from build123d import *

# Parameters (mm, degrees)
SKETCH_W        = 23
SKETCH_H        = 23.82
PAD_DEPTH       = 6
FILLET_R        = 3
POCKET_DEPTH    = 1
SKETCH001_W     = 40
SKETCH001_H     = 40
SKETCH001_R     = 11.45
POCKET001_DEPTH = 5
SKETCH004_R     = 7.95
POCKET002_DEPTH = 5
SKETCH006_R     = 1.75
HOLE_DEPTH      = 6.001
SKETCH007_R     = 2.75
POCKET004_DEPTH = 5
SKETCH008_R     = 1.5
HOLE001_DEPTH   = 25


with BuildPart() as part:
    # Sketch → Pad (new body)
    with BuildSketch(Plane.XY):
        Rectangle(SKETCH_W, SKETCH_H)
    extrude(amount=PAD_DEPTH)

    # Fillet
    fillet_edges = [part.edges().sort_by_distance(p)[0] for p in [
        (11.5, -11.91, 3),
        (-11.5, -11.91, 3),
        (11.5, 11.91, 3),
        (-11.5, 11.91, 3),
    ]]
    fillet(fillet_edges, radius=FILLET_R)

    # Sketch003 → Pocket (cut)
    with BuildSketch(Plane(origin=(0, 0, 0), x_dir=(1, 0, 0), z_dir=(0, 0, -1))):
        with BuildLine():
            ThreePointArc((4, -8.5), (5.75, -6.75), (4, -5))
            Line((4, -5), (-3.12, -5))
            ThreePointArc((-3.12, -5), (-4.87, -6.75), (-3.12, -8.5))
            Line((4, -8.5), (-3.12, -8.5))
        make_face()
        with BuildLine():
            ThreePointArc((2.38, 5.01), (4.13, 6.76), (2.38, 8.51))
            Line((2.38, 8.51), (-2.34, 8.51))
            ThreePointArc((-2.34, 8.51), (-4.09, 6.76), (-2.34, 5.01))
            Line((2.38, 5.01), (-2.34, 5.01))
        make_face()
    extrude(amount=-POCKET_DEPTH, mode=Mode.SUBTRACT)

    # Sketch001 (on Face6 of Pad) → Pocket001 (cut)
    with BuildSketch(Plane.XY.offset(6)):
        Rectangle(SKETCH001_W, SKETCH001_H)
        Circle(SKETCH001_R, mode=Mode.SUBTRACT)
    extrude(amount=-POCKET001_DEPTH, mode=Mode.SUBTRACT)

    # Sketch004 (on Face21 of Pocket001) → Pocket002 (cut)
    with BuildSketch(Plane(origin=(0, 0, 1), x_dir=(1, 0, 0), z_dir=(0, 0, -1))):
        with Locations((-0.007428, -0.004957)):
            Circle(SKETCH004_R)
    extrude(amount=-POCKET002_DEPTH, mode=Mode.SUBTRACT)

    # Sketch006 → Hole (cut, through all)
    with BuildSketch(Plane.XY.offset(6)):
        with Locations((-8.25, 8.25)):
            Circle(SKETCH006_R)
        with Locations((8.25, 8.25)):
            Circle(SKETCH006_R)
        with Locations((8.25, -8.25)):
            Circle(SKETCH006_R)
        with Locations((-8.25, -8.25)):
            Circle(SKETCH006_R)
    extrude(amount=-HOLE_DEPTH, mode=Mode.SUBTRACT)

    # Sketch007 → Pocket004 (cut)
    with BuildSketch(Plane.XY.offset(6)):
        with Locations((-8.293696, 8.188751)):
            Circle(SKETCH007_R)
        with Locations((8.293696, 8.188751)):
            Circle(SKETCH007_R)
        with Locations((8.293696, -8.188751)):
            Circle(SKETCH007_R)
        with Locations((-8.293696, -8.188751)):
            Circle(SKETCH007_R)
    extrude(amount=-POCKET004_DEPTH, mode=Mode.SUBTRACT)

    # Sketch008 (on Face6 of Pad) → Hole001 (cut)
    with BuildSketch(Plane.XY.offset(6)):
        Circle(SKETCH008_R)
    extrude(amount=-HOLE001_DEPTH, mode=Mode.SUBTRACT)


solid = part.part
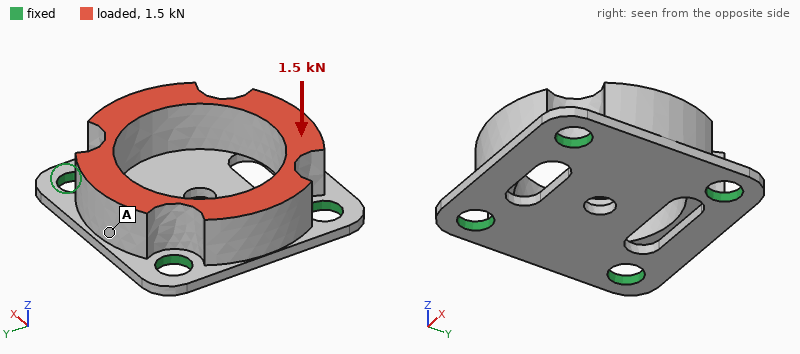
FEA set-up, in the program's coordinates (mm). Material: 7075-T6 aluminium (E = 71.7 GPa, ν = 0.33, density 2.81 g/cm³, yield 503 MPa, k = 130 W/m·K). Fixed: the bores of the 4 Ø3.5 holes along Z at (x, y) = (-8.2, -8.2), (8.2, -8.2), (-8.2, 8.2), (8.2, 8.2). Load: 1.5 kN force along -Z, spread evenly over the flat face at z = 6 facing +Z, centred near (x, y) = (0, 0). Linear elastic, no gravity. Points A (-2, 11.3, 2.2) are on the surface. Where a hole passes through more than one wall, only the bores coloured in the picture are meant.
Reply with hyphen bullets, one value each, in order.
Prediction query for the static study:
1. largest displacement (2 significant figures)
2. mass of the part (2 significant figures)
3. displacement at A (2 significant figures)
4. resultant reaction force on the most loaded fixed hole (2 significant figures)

- 8.0 µm
- 3.6 g
- 6.9 µm
- 400 N
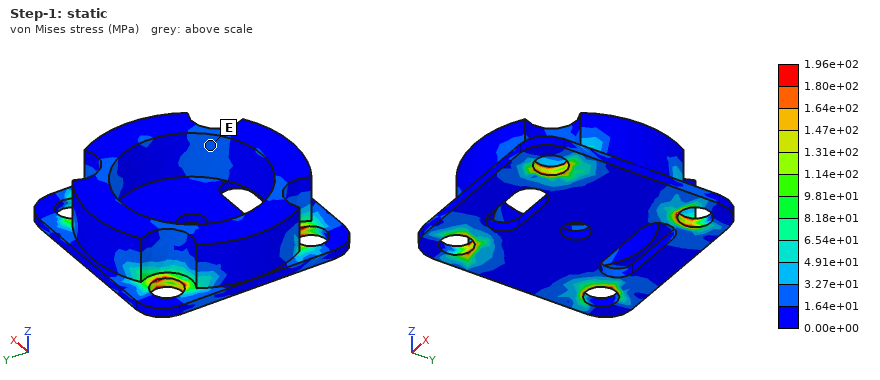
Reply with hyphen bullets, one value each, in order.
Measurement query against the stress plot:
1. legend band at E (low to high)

- 1.64e+01 to 3.27e+01 MPa
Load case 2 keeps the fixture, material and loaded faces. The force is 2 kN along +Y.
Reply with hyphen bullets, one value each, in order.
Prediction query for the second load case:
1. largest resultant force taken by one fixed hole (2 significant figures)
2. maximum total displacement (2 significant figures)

- 610 N
- 28 µm
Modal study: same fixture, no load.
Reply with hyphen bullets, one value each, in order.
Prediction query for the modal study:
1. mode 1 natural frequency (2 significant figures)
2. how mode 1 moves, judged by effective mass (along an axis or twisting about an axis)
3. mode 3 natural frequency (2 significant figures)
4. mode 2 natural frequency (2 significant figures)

- 25 kHz
- along Z
- 39 kHz
- 30 kHz
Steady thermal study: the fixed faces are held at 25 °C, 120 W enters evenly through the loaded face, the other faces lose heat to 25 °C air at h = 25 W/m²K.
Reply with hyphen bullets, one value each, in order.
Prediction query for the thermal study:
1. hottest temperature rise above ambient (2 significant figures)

- 82 K
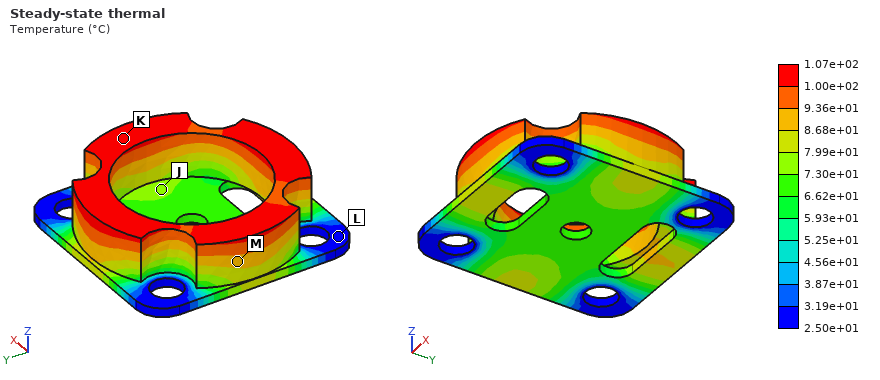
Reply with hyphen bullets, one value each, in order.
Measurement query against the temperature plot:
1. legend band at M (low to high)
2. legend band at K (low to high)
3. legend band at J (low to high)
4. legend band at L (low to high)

- 8.68e+01 to 9.36e+01 °C
- 1.00e+02 to 1.07e+02 °C
- 7.30e+01 to 7.99e+01 °C
- 2.50e+01 to 3.19e+01 °C
